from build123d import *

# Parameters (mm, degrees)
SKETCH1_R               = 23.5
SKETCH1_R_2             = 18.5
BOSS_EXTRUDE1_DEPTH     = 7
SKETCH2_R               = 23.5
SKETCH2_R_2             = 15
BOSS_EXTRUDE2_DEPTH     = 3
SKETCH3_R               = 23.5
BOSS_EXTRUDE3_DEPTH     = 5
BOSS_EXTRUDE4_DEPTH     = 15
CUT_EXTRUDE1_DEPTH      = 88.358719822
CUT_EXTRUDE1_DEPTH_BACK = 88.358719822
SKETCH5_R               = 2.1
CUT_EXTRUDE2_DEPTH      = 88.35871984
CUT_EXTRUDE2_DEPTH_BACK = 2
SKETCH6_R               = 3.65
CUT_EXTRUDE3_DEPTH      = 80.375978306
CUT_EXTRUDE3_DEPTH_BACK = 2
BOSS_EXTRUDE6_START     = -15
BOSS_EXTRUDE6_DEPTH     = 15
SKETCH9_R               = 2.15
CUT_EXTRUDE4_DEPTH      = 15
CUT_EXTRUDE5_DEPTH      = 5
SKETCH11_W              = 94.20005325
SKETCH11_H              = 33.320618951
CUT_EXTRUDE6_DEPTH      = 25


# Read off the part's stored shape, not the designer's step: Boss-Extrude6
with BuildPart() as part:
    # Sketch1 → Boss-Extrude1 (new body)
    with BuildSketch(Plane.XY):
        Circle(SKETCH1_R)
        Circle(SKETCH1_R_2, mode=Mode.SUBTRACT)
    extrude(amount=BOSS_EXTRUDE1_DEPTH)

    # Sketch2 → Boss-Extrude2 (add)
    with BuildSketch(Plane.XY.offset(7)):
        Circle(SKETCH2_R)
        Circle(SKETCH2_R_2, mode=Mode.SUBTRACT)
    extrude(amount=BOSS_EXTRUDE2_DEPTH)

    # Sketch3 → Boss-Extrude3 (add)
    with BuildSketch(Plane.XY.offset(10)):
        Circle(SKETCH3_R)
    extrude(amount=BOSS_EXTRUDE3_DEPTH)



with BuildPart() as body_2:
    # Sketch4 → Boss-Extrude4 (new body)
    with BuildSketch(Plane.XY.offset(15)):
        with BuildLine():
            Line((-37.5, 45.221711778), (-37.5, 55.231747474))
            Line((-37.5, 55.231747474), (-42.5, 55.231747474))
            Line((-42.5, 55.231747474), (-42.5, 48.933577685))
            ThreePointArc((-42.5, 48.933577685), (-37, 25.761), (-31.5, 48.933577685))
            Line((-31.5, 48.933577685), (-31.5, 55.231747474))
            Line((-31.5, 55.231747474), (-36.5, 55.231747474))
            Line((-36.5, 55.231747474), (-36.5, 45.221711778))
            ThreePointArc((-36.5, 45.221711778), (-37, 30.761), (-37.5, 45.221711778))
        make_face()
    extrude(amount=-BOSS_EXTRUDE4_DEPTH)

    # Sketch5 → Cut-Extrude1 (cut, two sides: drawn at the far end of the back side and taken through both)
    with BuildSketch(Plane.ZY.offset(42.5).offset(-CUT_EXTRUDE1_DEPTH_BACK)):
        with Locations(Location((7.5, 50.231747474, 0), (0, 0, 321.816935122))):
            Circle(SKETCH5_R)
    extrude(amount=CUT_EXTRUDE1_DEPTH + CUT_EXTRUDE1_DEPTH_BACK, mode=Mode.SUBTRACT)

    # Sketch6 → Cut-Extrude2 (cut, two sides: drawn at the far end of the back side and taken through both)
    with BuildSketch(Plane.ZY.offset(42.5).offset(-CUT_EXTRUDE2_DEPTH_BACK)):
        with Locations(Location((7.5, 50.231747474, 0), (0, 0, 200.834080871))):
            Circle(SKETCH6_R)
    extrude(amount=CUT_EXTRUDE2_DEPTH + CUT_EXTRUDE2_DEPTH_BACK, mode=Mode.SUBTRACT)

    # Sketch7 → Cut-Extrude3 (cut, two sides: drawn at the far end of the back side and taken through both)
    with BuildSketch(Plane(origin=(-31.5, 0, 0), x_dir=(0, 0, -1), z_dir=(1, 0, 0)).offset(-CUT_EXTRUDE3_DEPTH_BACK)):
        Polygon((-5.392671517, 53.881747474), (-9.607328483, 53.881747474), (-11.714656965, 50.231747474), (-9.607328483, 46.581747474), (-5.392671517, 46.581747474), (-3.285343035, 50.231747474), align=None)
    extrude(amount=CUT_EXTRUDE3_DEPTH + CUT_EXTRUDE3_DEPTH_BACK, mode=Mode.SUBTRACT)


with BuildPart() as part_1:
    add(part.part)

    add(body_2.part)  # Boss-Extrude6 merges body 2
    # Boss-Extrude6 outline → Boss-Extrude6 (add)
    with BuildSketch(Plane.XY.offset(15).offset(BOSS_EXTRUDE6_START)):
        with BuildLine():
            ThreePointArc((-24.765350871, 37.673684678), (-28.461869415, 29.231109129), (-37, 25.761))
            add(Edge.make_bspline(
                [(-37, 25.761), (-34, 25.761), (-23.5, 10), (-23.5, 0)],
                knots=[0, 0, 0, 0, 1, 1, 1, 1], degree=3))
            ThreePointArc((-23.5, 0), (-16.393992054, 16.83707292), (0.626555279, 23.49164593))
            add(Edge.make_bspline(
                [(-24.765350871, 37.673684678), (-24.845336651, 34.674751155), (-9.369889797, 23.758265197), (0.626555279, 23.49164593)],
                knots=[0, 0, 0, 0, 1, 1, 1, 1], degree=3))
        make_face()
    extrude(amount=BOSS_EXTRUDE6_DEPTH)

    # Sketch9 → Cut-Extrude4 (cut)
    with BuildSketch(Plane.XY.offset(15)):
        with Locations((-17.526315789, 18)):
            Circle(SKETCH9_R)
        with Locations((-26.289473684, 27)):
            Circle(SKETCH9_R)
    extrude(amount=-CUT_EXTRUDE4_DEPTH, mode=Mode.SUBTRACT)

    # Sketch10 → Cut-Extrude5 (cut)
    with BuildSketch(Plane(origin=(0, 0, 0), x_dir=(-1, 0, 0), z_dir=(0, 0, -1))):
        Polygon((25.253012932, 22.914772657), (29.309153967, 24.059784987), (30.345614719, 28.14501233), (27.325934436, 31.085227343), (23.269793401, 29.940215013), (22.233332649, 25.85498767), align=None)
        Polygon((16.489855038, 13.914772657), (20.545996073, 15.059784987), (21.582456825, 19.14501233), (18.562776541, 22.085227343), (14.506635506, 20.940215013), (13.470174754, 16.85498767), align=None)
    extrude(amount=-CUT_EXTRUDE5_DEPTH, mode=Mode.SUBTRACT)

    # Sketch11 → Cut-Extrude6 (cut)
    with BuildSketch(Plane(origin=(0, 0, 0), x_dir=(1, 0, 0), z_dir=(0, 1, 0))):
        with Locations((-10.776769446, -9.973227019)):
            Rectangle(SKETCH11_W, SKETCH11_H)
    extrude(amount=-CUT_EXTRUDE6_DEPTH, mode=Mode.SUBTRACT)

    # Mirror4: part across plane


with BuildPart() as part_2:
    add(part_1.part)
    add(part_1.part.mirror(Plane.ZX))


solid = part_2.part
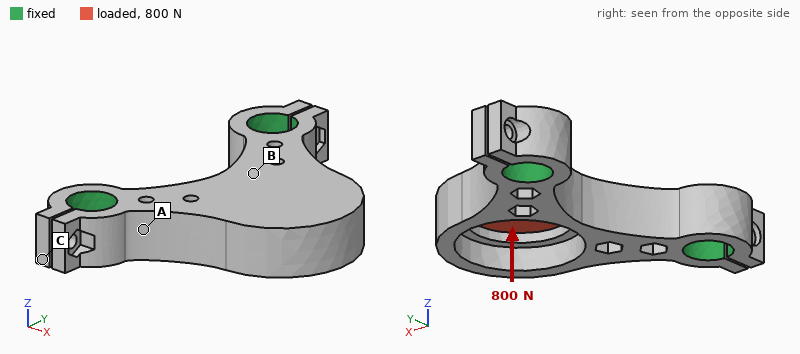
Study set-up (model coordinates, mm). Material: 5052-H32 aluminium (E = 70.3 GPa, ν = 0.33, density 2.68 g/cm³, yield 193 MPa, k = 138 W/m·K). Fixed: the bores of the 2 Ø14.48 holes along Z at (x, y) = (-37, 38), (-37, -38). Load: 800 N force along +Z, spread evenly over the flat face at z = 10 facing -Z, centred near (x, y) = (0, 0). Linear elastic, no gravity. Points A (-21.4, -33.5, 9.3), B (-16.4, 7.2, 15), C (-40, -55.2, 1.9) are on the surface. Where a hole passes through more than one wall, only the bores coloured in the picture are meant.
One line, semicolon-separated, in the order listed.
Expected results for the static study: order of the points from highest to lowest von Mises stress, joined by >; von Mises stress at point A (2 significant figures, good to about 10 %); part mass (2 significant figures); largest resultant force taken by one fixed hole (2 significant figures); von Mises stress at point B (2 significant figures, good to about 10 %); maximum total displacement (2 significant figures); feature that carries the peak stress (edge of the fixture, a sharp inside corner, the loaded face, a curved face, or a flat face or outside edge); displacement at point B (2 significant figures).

A > B > C; 17 MPa; 98 g; 400 N; 8.4 MPa; 68 µm; a curved face; 17 µm
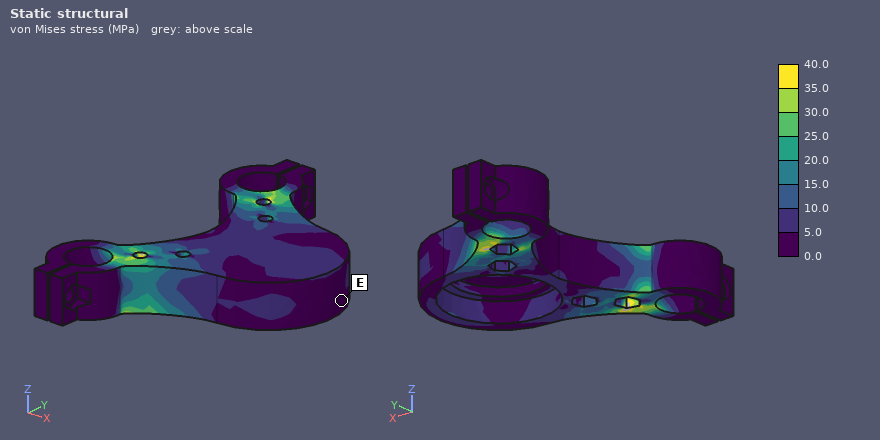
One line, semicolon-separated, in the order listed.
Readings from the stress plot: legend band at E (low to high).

0.0 to 5.0 MPa
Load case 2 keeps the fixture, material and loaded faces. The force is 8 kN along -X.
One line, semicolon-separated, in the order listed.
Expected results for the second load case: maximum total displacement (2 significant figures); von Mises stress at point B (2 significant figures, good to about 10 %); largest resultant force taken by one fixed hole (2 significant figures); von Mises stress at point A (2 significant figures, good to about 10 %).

51 µm; 27 MPa; 4.9 kN; 19 MPa
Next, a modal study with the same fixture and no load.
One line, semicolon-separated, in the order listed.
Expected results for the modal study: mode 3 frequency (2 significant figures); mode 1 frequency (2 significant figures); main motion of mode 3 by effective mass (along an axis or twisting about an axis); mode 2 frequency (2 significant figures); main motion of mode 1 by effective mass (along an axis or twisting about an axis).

12 kHz; 3200 Hz; along Z; 7800 Hz; along Z
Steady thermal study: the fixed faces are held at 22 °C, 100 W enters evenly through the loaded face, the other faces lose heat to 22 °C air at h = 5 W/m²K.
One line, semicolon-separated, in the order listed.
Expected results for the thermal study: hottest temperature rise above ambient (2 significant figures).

75 K
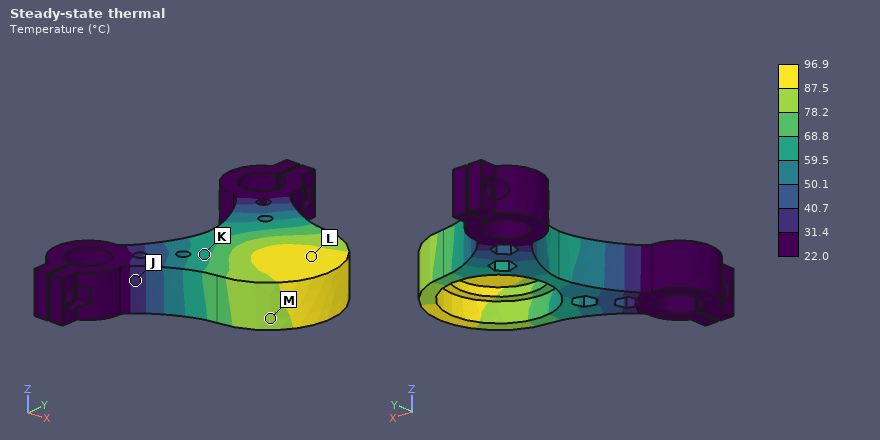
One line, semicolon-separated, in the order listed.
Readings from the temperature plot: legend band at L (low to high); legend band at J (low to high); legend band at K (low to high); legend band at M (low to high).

87.5 to 96.9 °C; 31.4 to 40.7 °C; 59.5 to 68.8 °C; 78.2 to 87.5 °C
